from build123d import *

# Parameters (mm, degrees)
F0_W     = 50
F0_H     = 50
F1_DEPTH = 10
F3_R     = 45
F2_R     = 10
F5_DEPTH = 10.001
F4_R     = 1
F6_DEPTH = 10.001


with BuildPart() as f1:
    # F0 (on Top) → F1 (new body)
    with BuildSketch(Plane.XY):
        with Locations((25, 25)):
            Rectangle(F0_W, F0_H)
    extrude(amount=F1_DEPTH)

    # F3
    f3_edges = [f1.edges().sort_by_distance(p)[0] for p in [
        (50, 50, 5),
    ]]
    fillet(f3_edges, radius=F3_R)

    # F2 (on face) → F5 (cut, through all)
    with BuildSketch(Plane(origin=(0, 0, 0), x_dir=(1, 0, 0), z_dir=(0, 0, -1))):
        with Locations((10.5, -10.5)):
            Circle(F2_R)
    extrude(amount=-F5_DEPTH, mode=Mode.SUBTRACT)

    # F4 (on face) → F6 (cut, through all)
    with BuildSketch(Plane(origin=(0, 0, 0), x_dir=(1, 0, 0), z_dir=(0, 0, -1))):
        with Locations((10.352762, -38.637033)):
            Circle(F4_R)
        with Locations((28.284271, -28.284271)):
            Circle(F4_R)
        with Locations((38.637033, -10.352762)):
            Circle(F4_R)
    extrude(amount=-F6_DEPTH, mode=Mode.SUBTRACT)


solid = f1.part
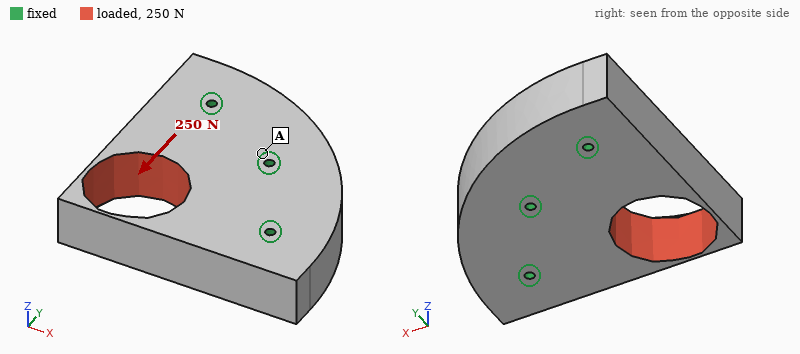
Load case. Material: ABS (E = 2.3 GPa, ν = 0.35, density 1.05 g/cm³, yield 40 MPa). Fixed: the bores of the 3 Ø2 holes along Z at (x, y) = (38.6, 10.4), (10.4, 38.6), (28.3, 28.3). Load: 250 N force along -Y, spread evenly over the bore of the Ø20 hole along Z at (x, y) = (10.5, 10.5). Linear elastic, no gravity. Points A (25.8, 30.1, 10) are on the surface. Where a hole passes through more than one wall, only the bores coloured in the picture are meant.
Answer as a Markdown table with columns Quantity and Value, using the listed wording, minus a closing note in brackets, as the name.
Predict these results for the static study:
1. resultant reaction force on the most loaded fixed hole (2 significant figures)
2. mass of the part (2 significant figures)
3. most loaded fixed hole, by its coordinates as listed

| Quantity | Value |
|---|---|
| resultant reaction force on the most loaded fixed hole | 170 N |
| mass of the part | 18 g |
| most loaded fixed hole, by its coordinates as listed | (10.4, 38.6) |
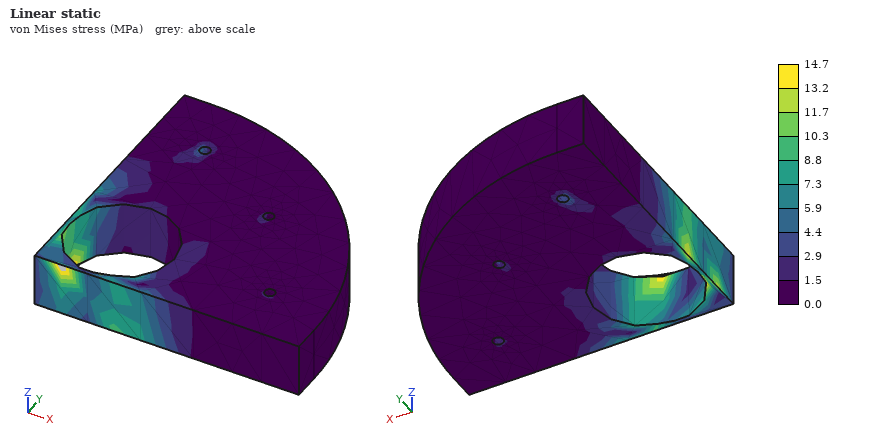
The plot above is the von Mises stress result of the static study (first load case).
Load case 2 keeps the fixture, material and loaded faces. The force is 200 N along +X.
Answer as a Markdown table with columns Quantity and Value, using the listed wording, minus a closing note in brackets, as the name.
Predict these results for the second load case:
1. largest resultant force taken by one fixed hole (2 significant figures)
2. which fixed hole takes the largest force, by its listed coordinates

| Quantity | Value |
|---|---|
| largest resultant force taken by one fixed hole | 140 N |
| which fixed hole takes the largest force, by its listed coordinates | (38.6, 10.4) |
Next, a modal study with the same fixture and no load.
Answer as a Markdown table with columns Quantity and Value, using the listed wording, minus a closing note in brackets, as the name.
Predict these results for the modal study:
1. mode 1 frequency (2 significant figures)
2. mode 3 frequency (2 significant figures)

| Quantity | Value |
|---|---|
| mode 1 frequency | 3100 Hz |
| mode 3 frequency | 5900 Hz |
